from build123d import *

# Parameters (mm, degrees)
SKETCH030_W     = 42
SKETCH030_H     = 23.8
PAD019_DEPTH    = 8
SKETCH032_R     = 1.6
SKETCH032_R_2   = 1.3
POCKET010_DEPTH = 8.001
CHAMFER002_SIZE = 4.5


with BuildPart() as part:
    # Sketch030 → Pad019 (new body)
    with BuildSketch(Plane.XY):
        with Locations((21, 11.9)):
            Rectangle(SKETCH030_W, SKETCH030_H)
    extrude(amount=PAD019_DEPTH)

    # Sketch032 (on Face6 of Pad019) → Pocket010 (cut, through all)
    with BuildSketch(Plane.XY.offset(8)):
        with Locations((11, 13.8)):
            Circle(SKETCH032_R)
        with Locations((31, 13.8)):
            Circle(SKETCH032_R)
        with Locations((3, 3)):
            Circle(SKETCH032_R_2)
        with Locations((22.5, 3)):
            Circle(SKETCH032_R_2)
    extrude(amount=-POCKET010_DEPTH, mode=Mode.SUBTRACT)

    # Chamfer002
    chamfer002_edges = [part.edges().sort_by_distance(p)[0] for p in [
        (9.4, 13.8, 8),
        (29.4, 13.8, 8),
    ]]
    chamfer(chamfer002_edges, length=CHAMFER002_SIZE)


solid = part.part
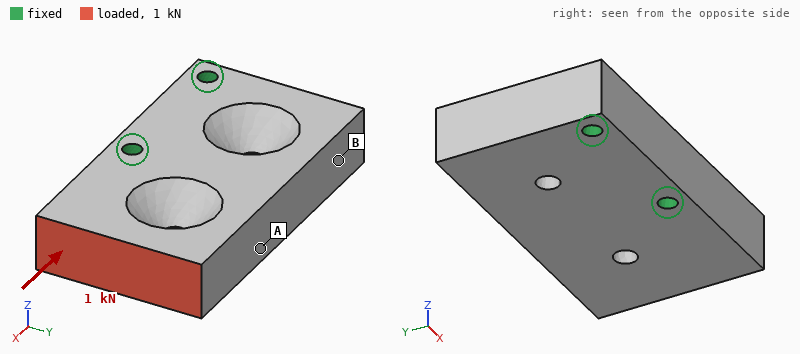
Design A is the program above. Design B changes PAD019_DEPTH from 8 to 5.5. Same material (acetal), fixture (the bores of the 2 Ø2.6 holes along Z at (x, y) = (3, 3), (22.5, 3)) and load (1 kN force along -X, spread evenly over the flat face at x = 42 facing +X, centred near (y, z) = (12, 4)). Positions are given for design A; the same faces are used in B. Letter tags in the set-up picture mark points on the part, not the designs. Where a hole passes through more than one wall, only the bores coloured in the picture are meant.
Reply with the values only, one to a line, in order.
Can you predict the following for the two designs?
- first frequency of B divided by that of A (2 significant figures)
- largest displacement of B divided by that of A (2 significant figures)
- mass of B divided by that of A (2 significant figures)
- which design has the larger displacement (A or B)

0.75
1.6
0.67
B
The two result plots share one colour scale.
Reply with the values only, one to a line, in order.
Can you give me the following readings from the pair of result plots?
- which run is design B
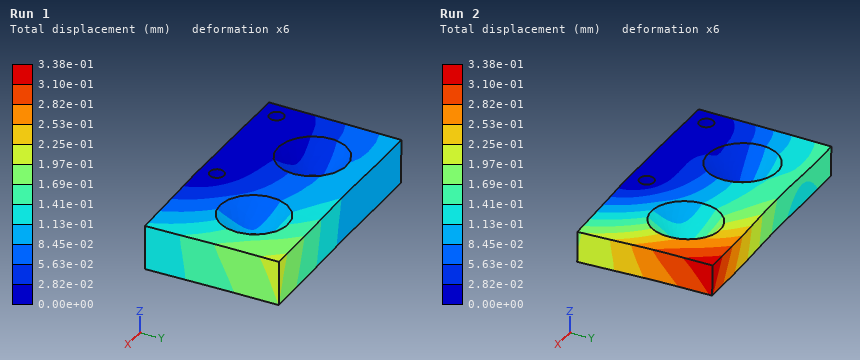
Run 2
